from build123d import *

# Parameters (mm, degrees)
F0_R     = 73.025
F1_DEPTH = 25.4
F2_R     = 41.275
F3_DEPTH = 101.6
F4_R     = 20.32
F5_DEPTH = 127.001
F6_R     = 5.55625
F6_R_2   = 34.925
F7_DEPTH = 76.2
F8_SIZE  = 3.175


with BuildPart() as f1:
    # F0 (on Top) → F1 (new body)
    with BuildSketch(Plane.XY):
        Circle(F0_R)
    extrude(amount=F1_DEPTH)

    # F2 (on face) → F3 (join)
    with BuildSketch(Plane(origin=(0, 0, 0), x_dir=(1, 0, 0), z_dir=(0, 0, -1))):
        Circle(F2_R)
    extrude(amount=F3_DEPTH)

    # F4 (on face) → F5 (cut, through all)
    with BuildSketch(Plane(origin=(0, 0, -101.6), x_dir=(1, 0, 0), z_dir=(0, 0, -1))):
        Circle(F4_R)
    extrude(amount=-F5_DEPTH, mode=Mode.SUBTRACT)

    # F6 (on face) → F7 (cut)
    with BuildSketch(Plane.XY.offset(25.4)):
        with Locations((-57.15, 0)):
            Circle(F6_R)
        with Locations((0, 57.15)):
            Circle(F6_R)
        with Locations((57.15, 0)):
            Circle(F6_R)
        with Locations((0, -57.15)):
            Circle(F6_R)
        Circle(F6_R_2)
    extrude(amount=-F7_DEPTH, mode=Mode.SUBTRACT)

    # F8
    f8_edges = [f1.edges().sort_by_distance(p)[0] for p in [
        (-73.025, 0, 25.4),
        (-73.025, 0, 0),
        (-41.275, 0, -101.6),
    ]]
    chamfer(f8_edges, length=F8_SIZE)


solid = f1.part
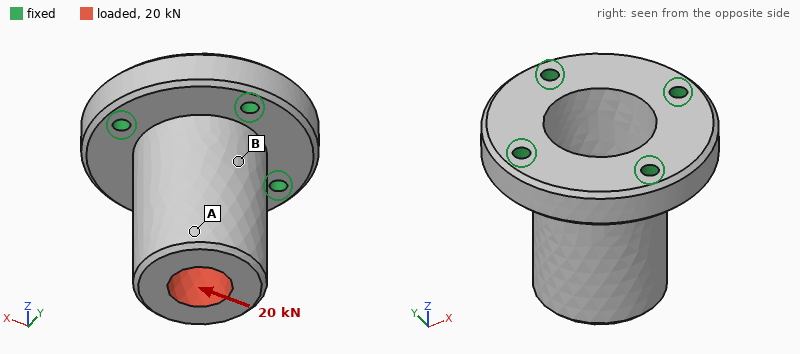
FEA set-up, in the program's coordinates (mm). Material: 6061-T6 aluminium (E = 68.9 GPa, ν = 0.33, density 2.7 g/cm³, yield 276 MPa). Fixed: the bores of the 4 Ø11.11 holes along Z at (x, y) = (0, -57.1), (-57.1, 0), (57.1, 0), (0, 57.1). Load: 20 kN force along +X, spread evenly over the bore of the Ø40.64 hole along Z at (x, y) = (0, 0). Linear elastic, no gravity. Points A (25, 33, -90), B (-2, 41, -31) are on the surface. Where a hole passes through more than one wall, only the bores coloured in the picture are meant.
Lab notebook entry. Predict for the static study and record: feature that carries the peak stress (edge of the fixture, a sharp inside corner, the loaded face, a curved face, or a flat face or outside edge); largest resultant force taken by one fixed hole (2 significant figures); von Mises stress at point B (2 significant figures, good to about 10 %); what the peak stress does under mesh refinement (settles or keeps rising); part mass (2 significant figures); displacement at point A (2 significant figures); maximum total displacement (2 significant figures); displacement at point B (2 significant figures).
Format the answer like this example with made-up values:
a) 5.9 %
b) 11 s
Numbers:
a) edge of the fixture
b) 17 kN
c) 40 MPa
d) keeps rising
e) 1.6 kg
f) 0.16 mm
g) 0.18 mm
h) 0.058 mm
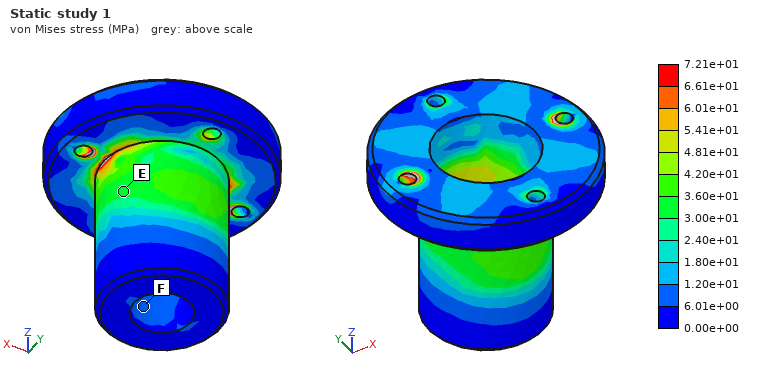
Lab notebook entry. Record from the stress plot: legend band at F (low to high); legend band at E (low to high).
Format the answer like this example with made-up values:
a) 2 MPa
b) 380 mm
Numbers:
a) 6.01e+00 to 1.20e+01 MPa
b) 3.00e+01 to 3.60e+01 MPa
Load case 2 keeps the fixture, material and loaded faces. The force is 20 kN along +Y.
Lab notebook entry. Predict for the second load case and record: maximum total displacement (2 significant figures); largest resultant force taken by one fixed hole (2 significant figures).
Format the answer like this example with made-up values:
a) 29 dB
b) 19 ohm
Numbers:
a) 0.18 mm
b) 17 kN
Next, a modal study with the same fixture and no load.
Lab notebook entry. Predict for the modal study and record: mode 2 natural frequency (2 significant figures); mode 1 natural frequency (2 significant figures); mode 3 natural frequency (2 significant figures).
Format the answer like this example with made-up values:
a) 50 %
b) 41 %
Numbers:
a) 2400 Hz
b) 2400 Hz
c) 5600 Hz
